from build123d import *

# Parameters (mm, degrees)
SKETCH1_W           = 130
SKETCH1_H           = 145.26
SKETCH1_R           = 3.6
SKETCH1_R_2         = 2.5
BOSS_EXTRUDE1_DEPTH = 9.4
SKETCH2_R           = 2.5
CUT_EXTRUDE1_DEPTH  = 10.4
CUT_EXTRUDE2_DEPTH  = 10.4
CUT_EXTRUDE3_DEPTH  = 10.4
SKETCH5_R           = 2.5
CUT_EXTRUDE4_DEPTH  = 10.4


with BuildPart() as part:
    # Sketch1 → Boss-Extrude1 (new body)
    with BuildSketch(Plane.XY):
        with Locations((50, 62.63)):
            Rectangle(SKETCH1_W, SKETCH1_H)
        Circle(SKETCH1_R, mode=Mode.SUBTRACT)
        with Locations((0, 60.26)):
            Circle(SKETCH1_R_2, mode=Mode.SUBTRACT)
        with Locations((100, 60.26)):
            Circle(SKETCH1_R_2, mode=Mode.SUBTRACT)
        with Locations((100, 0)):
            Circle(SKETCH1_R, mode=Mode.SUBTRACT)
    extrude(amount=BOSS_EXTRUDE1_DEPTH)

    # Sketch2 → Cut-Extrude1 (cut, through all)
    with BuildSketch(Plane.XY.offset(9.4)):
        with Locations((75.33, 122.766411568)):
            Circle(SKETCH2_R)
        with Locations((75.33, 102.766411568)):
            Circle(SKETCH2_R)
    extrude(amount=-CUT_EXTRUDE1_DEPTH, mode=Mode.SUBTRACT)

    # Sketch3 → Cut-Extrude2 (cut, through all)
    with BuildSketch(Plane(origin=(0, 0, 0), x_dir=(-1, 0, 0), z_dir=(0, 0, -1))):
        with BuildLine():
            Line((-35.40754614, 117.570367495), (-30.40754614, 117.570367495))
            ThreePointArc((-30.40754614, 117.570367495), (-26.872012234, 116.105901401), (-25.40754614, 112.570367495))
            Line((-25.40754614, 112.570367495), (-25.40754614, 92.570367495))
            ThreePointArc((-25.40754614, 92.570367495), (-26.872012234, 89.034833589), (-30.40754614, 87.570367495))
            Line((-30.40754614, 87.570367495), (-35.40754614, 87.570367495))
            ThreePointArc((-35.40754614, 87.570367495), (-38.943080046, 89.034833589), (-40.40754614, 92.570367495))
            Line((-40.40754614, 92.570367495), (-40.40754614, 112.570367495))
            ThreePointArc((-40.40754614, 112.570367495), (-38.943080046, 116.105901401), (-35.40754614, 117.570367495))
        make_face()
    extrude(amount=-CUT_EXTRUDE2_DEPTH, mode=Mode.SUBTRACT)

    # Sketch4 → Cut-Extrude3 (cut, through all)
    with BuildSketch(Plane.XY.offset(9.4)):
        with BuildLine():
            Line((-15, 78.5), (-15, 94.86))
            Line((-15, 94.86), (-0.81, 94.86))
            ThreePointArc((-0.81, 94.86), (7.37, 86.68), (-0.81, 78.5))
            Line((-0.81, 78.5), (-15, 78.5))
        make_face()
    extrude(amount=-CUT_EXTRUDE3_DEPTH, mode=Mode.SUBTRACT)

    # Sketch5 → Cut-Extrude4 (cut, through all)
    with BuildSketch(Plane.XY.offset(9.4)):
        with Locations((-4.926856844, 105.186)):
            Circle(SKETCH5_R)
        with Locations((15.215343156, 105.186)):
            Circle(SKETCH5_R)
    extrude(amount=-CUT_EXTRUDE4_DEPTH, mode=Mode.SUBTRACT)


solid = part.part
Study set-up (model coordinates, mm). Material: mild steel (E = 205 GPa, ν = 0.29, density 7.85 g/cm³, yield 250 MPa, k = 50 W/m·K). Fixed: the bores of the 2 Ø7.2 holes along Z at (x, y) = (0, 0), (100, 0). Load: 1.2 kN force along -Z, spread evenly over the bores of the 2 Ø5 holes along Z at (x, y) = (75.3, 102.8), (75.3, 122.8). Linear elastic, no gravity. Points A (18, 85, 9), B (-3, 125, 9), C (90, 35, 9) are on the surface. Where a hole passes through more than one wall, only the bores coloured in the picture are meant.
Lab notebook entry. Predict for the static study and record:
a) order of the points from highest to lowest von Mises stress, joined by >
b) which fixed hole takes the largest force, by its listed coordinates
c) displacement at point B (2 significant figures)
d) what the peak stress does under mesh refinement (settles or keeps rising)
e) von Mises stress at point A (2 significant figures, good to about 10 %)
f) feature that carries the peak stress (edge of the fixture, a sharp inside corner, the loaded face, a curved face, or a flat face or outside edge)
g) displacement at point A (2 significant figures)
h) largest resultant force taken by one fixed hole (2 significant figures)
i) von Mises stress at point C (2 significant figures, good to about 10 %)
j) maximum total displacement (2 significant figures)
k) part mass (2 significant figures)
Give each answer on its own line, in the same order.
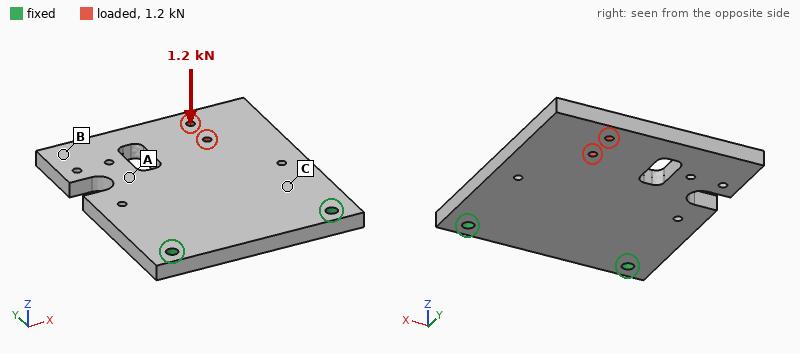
C > A > B
(100, 0)
0.43 mm
keeps rising
32 MPa
edge of the fixture
0.26 mm
890 N
54 MPa
0.59 mm
1.3 kg
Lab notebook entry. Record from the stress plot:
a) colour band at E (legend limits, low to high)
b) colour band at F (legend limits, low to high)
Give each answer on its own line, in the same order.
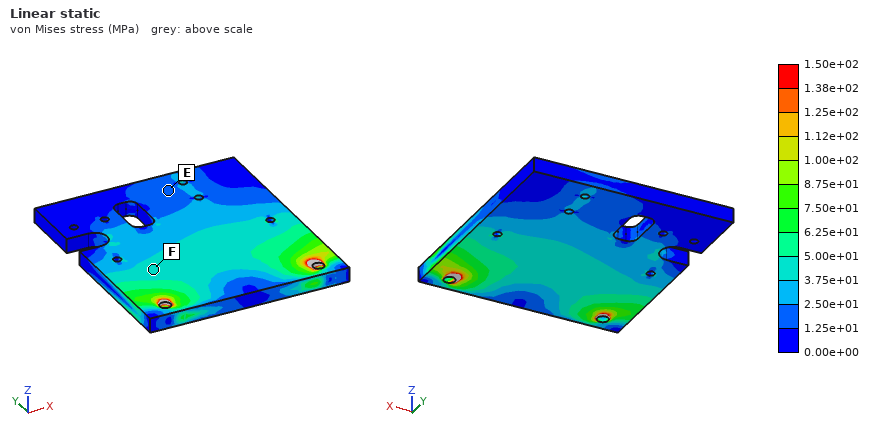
1.25e+01 to 2.50e+01 MPa
3.75e+01 to 5.00e+01 MPa
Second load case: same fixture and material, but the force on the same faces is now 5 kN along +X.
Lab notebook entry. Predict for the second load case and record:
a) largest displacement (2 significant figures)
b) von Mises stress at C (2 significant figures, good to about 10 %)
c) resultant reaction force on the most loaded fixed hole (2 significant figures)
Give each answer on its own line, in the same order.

23 µm
12 MPa
6.1 kN
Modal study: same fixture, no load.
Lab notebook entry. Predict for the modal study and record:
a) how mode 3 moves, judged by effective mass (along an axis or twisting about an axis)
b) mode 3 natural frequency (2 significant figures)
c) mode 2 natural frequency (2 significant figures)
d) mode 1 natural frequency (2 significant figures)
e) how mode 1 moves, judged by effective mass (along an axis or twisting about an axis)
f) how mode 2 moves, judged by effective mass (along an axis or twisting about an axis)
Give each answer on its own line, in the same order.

along Z
2200 Hz
1000 Hz
370 Hz
along Z
twisting about Y
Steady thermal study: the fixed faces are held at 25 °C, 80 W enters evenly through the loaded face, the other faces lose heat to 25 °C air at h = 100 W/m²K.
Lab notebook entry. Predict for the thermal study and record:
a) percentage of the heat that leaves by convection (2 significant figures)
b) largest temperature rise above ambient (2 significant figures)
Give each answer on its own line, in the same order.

92 %
84 K
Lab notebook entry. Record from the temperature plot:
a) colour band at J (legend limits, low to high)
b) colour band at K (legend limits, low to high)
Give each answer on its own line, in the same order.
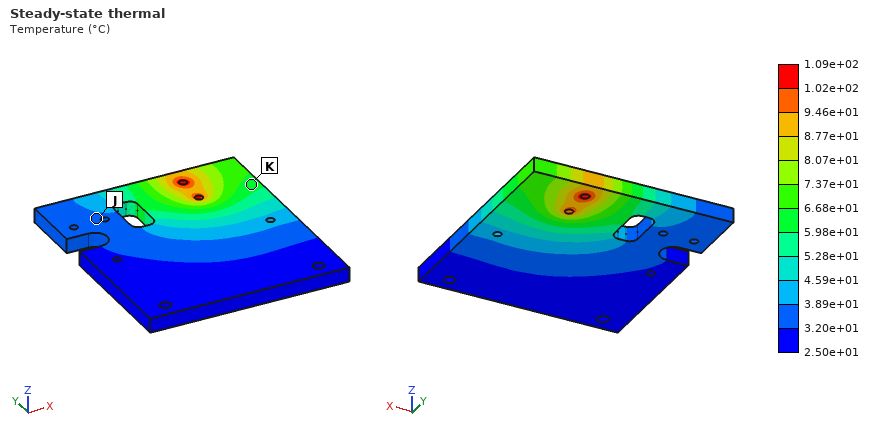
3.20e+01 to 3.89e+01 °C
5.98e+01 to 6.68e+01 °C
